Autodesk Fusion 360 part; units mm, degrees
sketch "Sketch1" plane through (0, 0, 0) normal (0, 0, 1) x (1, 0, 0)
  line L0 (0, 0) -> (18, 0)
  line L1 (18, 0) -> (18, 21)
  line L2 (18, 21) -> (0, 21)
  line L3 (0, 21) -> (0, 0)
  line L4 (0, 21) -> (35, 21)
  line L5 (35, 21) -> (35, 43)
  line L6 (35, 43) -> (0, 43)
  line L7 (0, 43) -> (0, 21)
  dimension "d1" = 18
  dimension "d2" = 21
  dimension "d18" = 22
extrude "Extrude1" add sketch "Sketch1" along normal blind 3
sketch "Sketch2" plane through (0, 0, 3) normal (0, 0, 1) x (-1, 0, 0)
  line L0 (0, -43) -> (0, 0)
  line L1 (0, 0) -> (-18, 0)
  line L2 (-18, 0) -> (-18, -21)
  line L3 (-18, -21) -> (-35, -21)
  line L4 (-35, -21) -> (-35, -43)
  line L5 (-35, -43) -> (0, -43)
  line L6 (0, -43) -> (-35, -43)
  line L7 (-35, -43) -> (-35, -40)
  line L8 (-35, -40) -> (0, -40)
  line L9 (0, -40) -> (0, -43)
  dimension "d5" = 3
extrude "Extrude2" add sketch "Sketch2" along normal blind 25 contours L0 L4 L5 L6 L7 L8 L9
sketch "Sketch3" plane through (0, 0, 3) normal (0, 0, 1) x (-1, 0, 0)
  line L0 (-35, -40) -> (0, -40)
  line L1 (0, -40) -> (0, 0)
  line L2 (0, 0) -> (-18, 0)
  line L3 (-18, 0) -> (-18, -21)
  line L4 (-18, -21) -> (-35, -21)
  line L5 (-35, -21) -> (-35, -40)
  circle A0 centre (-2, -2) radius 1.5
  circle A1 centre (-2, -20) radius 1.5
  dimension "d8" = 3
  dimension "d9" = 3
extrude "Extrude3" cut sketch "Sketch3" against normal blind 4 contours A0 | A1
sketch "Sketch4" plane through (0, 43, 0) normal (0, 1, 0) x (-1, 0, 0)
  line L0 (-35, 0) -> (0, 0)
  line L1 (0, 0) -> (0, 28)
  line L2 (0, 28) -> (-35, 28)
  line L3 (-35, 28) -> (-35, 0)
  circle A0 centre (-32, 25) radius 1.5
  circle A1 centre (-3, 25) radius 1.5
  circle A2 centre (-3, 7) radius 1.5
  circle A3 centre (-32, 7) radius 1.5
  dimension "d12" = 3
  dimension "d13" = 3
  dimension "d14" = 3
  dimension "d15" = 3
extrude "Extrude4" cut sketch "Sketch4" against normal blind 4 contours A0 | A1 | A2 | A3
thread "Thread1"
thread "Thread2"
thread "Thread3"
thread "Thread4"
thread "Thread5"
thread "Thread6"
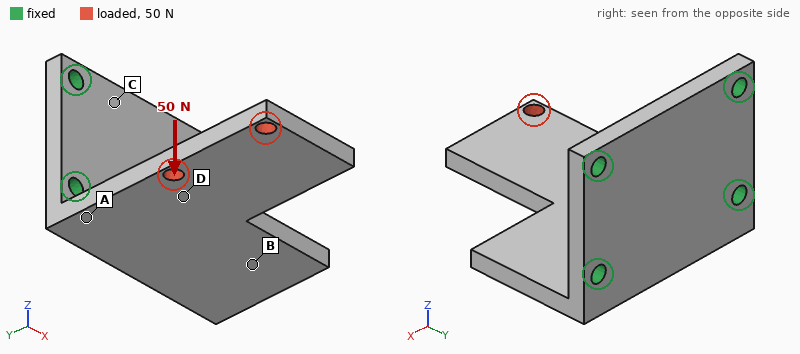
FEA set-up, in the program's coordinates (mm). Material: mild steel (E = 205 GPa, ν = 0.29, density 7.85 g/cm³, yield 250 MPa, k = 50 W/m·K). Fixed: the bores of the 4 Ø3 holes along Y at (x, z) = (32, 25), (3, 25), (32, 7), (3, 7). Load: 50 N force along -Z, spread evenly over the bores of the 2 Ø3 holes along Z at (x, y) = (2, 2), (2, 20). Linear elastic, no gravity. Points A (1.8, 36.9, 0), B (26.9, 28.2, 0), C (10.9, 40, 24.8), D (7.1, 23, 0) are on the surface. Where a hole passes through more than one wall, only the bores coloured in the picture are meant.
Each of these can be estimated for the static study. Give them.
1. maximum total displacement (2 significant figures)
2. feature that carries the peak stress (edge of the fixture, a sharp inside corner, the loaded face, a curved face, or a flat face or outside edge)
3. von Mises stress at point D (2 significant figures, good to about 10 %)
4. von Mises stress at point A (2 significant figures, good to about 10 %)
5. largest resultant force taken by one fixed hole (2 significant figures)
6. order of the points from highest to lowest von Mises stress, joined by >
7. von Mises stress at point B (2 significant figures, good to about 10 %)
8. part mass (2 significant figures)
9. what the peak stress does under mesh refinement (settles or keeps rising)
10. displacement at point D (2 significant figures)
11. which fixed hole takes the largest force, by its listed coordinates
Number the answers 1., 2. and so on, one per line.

1. 93 µm
2. edge of the fixture
3. 23 MPa
4. 36 MPa
5. 43 N
6. A > D > B > C
7. 15 MPa
8. 47 g
9. keeps rising
10. 27 µm
11. (3, 7)
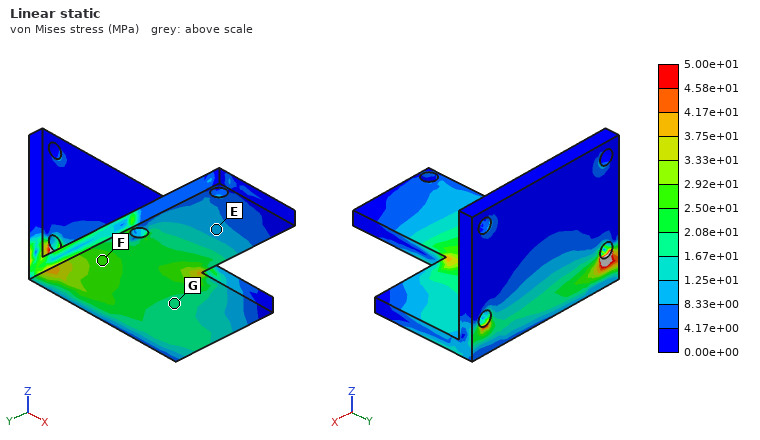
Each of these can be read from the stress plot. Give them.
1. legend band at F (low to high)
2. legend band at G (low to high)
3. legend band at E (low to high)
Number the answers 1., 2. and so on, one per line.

1. 2.50e+01 to 2.92e+01 MPa
2. 1.67e+01 to 2.08e+01 MPa
3. 8.33e+00 to 1.25e+01 MPa
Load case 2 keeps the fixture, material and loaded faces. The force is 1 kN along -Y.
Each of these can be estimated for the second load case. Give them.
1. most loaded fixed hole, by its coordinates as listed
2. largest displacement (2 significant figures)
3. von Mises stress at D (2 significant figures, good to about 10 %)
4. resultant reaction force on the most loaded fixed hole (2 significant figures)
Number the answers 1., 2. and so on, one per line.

1. (3, 7)
2. 66 µm
3. 30 MPa
4. 1.1 kN
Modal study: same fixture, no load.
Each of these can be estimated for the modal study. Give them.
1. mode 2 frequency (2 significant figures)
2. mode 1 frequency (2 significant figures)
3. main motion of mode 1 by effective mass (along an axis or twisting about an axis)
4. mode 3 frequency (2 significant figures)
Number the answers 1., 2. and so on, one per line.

1. 5900 Hz
2. 1500 Hz
3. along Z
4. 7100 Hz
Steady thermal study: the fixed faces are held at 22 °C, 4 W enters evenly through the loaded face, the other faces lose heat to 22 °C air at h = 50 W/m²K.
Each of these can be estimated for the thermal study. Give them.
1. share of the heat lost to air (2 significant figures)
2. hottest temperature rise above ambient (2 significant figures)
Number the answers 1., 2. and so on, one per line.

1. 45 %
2. 42 K
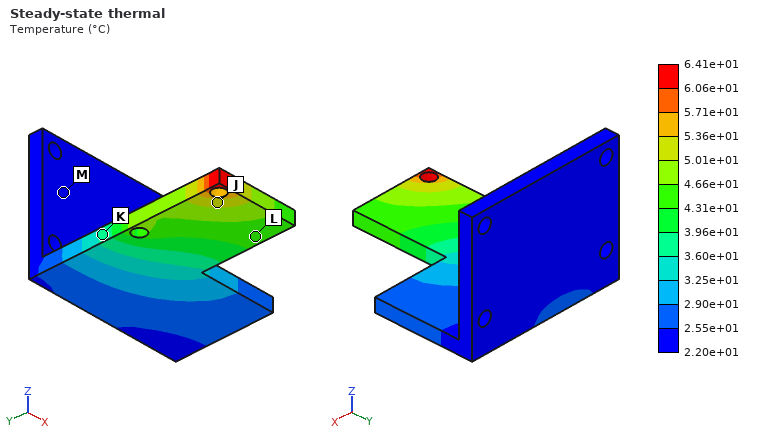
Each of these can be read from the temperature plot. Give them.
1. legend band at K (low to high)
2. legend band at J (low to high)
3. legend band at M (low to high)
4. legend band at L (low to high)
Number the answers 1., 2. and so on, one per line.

1. 3.60e+01 to 3.96e+01 °C
2. 5.01e+01 to 5.36e+01 °C
3. 2.20e+01 to 2.55e+01 °C
4. 4.31e+01 to 4.66e+01 °C
